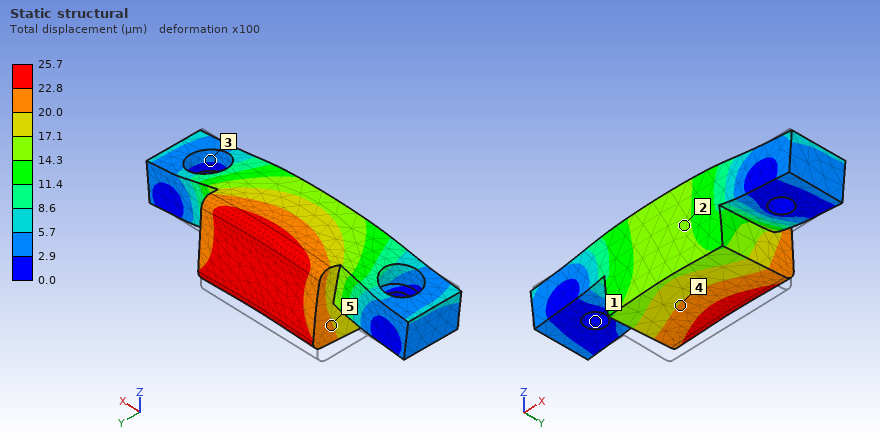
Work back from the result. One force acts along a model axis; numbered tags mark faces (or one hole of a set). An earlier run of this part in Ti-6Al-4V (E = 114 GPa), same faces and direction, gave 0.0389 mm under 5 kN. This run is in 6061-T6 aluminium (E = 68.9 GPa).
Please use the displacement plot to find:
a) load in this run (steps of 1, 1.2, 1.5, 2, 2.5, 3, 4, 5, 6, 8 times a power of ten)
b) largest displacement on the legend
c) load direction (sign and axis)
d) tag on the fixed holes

2 kN
25.7 µm
+Z
1
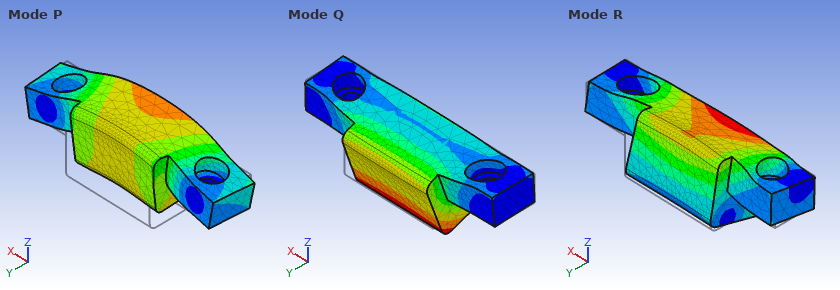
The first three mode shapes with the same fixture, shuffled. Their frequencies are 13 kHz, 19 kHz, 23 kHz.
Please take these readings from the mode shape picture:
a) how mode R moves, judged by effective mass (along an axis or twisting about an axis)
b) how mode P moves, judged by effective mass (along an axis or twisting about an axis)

along Y
along Z
